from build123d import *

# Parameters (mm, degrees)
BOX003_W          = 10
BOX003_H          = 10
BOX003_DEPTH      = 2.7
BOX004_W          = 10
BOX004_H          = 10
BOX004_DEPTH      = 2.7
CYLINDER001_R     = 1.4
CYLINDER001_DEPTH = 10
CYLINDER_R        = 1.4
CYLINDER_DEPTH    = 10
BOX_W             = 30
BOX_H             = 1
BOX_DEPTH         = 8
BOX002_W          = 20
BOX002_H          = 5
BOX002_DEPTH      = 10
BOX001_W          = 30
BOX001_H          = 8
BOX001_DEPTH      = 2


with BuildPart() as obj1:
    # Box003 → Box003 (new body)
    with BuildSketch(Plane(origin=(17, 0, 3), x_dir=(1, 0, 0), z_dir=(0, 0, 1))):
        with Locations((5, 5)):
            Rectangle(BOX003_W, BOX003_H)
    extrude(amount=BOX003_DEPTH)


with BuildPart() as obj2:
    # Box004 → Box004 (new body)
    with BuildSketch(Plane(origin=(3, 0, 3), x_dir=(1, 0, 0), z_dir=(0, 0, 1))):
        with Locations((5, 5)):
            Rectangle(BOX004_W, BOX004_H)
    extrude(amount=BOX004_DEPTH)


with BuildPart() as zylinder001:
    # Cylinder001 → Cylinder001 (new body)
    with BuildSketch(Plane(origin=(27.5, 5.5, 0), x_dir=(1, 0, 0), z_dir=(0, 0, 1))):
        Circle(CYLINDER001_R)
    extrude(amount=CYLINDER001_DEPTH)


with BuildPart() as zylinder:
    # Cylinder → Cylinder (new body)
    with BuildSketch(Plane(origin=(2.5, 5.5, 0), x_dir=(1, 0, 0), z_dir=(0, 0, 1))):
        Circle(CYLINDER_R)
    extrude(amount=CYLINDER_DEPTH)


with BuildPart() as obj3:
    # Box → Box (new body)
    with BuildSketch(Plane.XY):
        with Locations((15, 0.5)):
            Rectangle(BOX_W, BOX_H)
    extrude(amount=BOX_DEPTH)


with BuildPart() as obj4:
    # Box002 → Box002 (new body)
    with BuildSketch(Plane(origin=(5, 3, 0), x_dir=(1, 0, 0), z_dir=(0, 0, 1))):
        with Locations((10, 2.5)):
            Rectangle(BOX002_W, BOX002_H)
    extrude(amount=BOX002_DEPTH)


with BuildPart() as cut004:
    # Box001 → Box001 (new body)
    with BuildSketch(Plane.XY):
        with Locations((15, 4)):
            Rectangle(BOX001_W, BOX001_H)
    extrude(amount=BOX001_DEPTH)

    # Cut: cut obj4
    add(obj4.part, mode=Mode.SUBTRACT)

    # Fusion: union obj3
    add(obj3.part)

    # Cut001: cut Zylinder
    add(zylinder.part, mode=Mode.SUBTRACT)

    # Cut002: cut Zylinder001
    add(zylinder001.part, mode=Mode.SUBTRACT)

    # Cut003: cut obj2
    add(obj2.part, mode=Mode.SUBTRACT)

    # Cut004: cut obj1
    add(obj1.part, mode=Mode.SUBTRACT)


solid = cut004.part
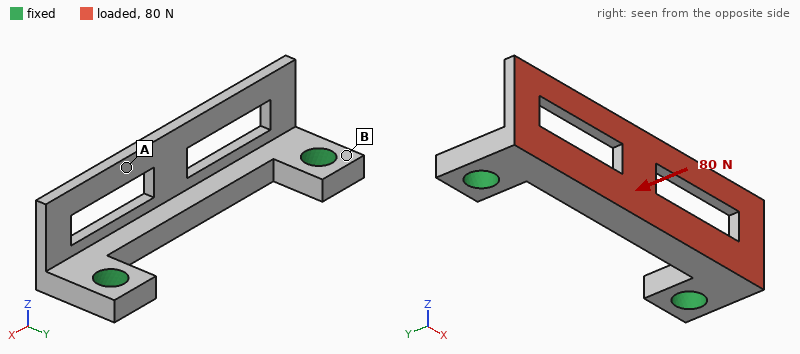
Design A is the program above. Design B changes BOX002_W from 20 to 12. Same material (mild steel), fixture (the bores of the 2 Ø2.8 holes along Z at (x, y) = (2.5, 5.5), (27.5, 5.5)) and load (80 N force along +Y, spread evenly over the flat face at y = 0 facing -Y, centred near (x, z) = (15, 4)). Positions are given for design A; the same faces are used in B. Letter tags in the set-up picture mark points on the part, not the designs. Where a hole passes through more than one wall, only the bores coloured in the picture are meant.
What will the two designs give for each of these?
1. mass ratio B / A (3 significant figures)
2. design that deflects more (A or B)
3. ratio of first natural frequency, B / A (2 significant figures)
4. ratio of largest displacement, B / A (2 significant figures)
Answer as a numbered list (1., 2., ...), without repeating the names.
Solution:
1. 1.21
2. A
3. 1.1
4. 0.83
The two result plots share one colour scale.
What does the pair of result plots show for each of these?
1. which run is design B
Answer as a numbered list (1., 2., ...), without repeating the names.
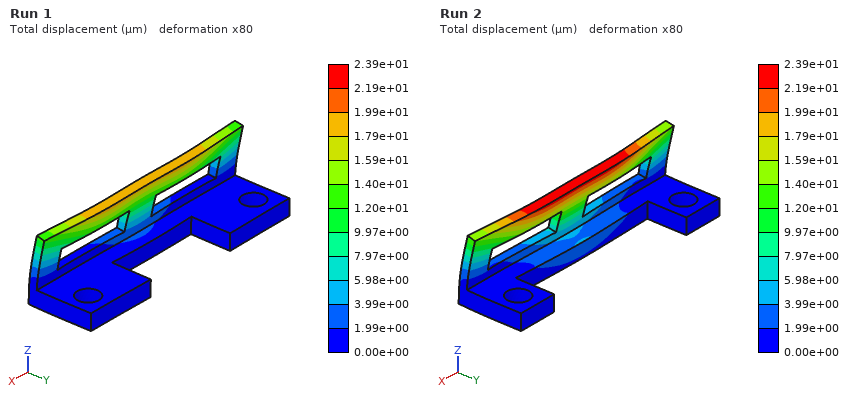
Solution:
1. Run 1
